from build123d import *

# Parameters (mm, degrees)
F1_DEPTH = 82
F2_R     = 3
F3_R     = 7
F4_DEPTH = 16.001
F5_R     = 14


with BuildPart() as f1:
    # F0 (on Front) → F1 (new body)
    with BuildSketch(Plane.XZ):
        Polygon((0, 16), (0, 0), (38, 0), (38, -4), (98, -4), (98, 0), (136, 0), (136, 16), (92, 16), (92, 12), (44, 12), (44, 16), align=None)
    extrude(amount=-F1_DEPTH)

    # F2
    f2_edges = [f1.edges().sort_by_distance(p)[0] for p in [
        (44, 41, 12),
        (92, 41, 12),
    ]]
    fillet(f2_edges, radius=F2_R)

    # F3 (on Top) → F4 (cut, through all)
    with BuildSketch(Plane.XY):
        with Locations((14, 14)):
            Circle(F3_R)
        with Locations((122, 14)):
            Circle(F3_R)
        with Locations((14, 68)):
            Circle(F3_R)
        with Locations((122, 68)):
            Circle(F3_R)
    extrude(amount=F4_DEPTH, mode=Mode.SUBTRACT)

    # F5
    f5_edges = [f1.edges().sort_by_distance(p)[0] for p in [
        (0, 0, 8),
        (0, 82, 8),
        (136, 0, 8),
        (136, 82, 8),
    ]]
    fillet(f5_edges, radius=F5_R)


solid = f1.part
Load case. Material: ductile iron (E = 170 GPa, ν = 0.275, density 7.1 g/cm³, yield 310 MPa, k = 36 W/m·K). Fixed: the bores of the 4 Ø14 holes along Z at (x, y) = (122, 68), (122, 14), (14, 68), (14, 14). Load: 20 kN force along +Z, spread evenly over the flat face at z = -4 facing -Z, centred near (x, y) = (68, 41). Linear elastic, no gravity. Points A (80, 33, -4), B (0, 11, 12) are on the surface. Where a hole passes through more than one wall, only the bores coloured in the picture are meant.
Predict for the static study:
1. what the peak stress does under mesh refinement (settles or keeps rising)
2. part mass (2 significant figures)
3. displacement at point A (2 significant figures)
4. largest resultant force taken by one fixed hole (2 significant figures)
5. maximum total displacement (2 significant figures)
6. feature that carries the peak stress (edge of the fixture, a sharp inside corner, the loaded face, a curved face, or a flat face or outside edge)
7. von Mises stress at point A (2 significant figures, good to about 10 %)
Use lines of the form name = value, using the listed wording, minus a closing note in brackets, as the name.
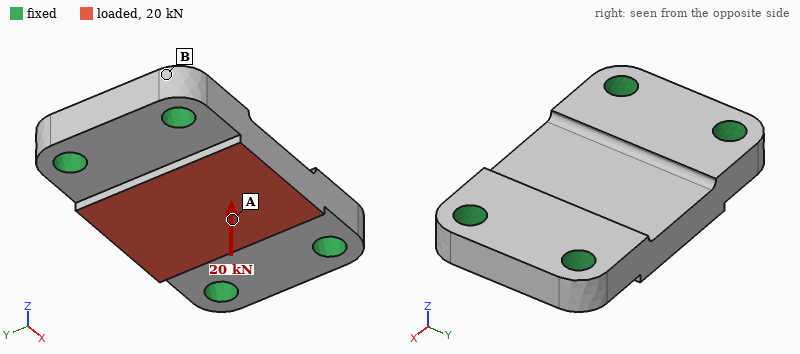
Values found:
what the peak stress does under mesh refinement = keeps rising
part mass = 1.2 kg
displacement at point A = 19 µm
largest resultant force taken by one fixed hole = 6.4 kN
maximum total displacement = 22 µm
feature that carries the peak stress = edge of the fixture
von Mises stress at point A = 29 MPa
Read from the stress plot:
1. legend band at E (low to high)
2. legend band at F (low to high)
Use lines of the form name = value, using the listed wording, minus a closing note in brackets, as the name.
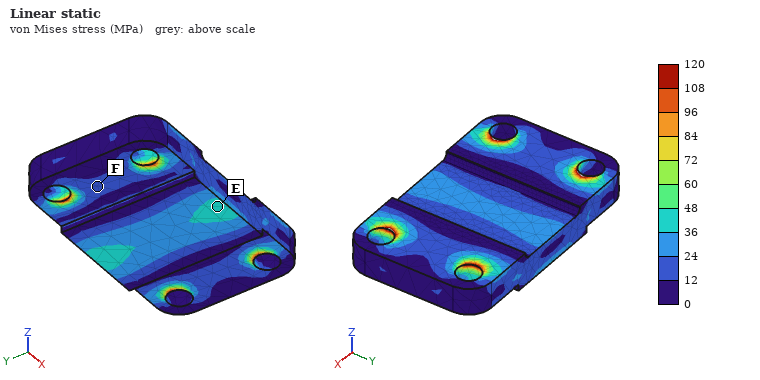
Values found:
legend band at E = 36 to 48 MPa
legend band at F = 12 to 24 MPa
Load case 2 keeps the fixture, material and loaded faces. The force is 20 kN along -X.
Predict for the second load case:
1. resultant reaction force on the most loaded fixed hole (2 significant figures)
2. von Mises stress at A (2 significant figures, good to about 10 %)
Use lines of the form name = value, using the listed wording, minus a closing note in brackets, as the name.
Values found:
resultant reaction force on the most loaded fixed hole = 5.3 kN
von Mises stress at A = 7.4 MPa
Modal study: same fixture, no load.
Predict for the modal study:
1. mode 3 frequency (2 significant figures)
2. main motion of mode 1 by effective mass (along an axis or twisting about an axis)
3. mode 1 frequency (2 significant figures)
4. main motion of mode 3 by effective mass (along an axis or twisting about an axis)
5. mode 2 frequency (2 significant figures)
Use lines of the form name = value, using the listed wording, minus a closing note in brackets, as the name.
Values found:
mode 3 frequency = 13 kHz
main motion of mode 1 by effective mass = along Z
mode 1 frequency = 6800 Hz
main motion of mode 3 by effective mass = along Y
mode 2 frequency = 8700 Hz
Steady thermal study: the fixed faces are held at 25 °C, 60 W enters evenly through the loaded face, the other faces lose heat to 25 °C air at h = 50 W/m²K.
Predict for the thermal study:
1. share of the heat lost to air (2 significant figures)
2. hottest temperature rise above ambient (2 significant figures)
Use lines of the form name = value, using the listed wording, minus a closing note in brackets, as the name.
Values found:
share of the heat lost to air = 17 %
hottest temperature rise above ambient = 24 K
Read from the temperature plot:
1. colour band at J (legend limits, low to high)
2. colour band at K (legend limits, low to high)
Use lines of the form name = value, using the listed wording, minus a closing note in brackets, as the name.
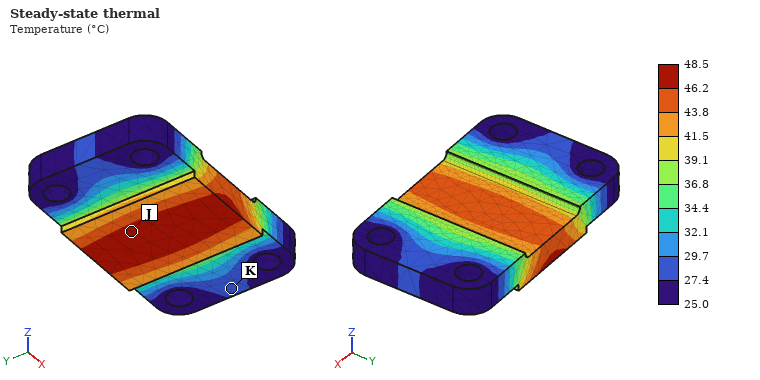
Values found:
colour band at J = 46.2 to 48.5 °C
colour band at K = 27.4 to 29.7 °C
